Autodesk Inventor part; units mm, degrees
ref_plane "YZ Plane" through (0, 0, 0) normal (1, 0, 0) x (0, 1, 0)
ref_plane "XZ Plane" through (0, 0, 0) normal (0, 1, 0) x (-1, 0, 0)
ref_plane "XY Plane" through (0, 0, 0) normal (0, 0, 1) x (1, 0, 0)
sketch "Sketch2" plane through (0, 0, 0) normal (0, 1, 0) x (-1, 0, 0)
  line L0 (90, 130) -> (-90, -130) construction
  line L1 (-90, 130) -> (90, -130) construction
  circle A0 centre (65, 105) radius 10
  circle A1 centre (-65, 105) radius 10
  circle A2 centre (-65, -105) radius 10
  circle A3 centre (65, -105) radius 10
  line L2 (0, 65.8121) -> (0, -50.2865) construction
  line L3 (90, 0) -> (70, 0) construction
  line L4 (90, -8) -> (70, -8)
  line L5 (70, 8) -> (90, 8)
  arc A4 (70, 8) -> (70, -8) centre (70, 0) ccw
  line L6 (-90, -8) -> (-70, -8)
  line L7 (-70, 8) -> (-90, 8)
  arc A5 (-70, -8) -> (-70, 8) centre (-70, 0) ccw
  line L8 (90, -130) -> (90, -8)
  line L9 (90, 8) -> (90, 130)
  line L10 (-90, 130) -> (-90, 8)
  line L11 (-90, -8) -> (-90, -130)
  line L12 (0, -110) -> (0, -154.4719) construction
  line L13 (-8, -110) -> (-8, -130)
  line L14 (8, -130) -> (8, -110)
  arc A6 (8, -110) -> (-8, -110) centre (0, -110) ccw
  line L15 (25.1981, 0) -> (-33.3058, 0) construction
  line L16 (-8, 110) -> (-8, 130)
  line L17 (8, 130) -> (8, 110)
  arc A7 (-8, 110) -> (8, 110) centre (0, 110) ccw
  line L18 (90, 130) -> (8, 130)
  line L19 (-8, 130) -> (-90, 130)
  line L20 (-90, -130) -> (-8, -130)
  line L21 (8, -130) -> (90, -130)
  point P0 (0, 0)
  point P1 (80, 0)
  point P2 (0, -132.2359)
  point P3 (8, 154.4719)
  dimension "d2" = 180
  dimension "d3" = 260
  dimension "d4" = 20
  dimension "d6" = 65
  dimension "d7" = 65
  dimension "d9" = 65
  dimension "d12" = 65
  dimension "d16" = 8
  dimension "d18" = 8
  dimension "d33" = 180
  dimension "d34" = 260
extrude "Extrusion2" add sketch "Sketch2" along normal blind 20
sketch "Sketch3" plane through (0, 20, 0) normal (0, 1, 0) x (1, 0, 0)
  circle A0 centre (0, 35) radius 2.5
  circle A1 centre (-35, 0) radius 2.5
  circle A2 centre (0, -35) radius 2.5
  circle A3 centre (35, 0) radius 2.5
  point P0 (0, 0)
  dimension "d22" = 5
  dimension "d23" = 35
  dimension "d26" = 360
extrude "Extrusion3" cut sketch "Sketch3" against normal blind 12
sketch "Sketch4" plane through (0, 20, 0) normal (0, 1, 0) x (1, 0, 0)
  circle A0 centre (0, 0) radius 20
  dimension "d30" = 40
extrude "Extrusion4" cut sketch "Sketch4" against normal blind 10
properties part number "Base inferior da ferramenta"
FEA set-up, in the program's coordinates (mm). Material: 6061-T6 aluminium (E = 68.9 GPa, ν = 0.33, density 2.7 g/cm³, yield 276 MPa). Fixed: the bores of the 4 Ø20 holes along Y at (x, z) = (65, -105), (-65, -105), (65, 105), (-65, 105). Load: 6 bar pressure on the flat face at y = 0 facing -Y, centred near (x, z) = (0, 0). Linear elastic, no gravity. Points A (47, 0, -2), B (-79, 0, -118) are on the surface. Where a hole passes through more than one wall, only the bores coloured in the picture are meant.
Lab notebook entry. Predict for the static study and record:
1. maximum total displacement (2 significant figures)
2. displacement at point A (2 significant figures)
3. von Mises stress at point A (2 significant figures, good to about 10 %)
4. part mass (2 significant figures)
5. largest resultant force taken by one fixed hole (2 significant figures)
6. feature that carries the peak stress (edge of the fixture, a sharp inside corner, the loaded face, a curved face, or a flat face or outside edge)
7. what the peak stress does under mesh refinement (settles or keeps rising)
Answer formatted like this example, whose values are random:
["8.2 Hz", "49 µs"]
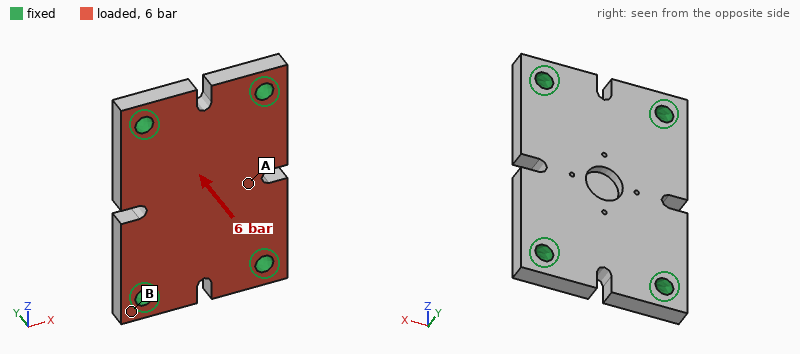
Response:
["95 µm", "88 µm", "22 MPa", "2.3 kg", "6.6 kN", "edge of the fixture", "keeps rising"]
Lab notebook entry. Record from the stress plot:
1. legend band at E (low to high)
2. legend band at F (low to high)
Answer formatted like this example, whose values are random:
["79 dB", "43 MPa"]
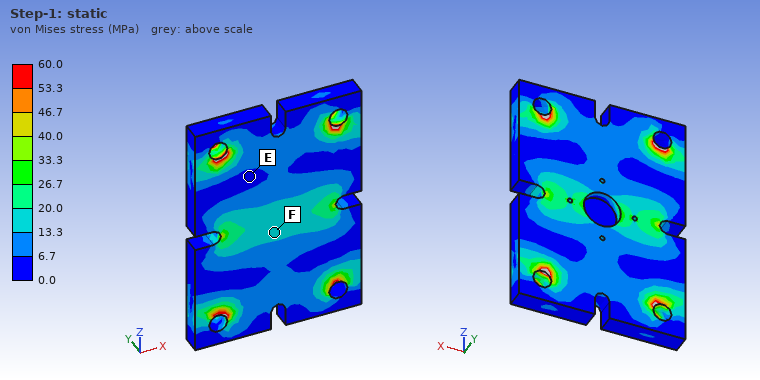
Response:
["0.0 to 6.7 MPa", "13.3 to 20.0 MPa"]
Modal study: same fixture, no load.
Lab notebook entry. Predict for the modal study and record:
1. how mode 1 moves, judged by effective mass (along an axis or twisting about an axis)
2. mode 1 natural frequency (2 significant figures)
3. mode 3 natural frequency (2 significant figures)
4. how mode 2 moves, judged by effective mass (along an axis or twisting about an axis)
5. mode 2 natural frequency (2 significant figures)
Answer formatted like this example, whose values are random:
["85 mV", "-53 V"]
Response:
["along Y", "2100 Hz", "4700 Hz", "twisting about Z", "2900 Hz"]
